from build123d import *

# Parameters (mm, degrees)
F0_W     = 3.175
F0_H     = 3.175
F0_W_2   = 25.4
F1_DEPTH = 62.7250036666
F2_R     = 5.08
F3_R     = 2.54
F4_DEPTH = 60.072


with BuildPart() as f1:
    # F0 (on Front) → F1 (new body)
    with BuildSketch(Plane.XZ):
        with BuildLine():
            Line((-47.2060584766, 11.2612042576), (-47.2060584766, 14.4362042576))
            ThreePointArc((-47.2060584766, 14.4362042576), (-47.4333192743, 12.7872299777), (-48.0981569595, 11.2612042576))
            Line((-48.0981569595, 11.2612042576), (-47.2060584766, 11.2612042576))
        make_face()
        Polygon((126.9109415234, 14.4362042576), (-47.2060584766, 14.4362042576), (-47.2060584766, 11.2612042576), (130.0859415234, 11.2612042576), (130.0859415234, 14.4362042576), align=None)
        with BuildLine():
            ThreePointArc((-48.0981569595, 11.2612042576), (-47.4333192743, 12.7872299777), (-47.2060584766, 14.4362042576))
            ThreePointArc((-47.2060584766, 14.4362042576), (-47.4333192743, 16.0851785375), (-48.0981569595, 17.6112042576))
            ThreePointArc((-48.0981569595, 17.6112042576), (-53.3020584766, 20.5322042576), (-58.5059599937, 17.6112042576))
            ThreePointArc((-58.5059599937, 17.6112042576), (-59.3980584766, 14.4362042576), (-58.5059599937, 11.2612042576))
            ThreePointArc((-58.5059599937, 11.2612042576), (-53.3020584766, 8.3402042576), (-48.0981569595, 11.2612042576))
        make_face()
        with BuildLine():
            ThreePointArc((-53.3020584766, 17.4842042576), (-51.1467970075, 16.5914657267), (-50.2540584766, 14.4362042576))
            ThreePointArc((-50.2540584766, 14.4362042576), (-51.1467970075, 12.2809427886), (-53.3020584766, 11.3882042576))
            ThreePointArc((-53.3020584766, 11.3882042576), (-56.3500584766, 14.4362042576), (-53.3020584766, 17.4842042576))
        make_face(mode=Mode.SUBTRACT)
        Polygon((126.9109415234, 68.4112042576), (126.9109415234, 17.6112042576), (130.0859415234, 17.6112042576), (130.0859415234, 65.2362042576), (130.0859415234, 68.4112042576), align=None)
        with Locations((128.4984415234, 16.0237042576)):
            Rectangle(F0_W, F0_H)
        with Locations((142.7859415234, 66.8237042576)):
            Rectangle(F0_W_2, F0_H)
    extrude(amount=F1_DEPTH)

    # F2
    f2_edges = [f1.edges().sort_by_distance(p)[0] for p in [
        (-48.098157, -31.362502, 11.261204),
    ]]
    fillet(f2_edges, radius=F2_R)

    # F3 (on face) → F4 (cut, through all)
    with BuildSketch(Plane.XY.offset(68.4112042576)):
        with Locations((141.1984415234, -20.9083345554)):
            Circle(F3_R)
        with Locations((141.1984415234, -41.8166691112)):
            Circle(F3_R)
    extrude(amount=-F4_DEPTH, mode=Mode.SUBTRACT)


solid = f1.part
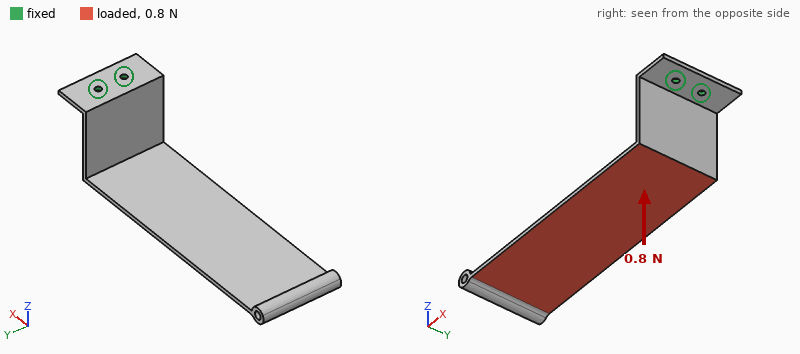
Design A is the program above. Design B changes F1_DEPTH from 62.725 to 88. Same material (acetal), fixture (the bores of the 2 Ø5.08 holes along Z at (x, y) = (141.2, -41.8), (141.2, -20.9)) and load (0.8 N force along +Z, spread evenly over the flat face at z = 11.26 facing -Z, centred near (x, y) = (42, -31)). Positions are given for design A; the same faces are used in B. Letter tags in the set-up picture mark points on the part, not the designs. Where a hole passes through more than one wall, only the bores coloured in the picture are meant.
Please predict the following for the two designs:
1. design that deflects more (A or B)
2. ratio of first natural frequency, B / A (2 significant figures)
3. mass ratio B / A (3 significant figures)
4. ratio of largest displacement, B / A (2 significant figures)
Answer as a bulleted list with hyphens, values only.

- A
- 0.98
- 1.40
- 0.74
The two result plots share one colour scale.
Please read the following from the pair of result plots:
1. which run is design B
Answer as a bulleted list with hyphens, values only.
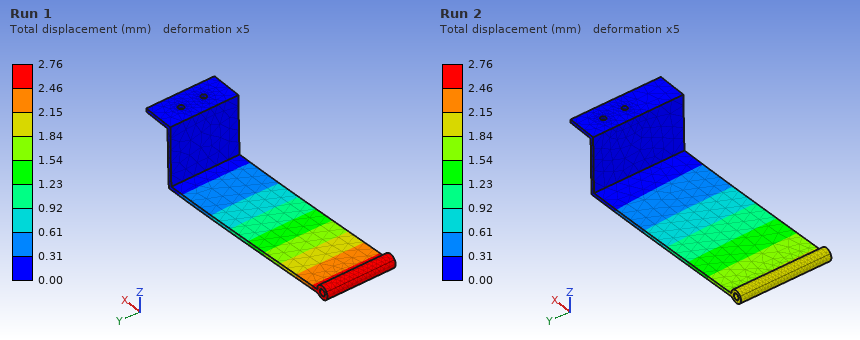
- Run 2
